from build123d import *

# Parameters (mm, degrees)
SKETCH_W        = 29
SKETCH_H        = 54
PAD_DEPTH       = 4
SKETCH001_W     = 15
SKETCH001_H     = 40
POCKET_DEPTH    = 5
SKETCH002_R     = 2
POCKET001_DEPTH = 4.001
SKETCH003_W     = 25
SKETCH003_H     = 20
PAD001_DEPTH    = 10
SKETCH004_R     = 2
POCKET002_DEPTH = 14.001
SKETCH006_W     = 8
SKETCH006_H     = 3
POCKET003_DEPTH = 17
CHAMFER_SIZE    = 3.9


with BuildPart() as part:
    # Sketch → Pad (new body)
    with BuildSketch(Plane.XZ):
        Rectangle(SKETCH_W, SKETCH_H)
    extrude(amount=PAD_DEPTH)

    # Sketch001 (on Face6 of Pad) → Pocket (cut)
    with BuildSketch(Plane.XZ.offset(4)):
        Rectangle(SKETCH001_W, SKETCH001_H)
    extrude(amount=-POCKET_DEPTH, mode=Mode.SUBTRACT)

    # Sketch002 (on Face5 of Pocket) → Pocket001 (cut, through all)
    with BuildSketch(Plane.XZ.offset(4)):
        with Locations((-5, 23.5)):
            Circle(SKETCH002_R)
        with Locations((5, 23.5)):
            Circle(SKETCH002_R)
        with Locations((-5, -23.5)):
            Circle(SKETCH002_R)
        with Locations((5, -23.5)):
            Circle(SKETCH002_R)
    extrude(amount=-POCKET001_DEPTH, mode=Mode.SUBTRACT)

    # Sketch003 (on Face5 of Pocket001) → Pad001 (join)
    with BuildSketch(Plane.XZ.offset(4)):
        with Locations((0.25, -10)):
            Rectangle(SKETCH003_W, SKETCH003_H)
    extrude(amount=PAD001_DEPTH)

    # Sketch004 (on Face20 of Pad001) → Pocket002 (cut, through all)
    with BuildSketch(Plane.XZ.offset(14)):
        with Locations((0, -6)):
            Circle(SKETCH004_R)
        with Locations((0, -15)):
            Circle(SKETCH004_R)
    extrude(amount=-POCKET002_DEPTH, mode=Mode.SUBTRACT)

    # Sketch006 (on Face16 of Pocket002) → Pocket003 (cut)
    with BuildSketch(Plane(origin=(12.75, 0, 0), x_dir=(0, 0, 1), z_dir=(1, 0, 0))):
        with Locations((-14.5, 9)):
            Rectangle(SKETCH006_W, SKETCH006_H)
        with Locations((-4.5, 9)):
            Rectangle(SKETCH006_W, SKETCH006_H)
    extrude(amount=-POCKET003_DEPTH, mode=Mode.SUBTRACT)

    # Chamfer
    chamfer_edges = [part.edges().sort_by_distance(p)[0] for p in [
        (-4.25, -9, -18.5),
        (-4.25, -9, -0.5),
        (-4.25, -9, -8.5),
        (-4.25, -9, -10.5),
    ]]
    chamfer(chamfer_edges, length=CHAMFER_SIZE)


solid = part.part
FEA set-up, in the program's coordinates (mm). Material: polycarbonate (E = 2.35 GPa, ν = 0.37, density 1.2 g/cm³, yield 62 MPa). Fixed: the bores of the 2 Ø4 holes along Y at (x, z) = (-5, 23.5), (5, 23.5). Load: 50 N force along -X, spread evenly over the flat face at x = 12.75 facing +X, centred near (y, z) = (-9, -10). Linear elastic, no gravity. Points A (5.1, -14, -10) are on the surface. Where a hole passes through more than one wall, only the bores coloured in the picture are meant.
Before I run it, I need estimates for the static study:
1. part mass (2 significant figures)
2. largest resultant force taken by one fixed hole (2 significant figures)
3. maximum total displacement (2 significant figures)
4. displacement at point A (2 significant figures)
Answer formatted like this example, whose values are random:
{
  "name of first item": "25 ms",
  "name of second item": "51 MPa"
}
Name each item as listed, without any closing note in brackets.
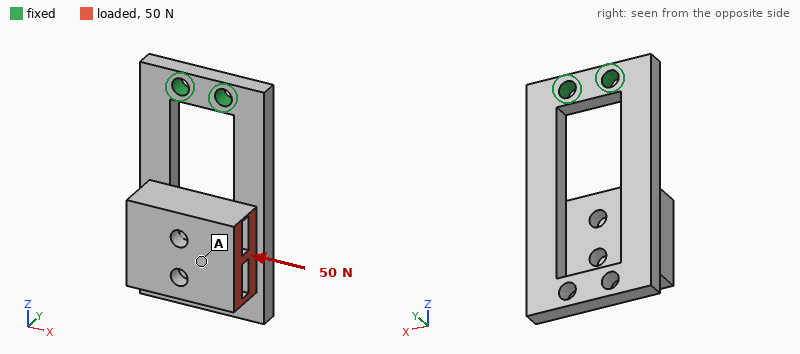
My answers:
{
  "part mass": "9.3 g",
  "largest resultant force taken by one fixed hole": "66 N",
  "maximum total displacement": "0.75 mm",
  "displacement at point A": "0.66 mm"
}
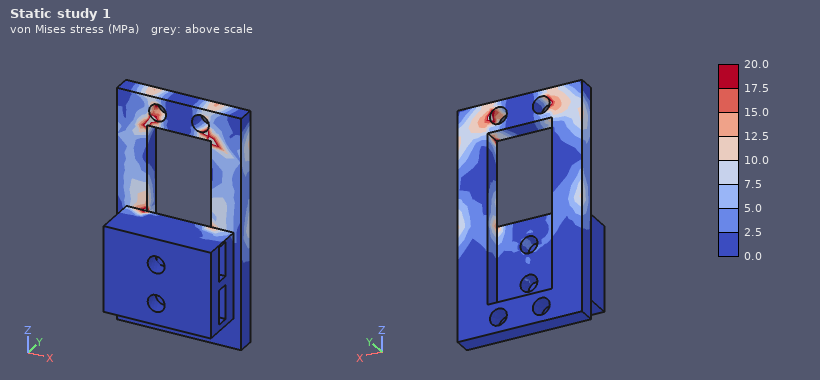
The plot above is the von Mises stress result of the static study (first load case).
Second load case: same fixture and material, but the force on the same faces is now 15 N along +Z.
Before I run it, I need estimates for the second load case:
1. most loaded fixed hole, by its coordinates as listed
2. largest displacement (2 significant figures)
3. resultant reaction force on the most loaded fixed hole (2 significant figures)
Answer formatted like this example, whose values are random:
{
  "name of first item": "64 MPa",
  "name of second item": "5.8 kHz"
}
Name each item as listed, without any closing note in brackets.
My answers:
{
  "most loaded fixed hole, by its coordinates as listed": "(5, 23.5)",
  "largest displacement": "0.63 mm",
  "resultant reaction force on the most loaded fixed hole": "17 N"
}
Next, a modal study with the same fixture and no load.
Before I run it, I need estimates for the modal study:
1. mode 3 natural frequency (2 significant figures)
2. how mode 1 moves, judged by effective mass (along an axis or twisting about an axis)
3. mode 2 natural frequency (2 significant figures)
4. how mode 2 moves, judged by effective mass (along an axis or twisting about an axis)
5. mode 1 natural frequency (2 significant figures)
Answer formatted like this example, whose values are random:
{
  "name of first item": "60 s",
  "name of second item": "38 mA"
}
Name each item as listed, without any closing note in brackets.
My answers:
{
  "mode 3 natural frequency": "790 Hz",
  "how mode 1 moves, judged by effective mass": "along Y",
  "mode 2 natural frequency": "550 Hz",
  "how mode 2 moves, judged by effective mass": "along X",
  "mode 1 natural frequency": "180 Hz"
}
